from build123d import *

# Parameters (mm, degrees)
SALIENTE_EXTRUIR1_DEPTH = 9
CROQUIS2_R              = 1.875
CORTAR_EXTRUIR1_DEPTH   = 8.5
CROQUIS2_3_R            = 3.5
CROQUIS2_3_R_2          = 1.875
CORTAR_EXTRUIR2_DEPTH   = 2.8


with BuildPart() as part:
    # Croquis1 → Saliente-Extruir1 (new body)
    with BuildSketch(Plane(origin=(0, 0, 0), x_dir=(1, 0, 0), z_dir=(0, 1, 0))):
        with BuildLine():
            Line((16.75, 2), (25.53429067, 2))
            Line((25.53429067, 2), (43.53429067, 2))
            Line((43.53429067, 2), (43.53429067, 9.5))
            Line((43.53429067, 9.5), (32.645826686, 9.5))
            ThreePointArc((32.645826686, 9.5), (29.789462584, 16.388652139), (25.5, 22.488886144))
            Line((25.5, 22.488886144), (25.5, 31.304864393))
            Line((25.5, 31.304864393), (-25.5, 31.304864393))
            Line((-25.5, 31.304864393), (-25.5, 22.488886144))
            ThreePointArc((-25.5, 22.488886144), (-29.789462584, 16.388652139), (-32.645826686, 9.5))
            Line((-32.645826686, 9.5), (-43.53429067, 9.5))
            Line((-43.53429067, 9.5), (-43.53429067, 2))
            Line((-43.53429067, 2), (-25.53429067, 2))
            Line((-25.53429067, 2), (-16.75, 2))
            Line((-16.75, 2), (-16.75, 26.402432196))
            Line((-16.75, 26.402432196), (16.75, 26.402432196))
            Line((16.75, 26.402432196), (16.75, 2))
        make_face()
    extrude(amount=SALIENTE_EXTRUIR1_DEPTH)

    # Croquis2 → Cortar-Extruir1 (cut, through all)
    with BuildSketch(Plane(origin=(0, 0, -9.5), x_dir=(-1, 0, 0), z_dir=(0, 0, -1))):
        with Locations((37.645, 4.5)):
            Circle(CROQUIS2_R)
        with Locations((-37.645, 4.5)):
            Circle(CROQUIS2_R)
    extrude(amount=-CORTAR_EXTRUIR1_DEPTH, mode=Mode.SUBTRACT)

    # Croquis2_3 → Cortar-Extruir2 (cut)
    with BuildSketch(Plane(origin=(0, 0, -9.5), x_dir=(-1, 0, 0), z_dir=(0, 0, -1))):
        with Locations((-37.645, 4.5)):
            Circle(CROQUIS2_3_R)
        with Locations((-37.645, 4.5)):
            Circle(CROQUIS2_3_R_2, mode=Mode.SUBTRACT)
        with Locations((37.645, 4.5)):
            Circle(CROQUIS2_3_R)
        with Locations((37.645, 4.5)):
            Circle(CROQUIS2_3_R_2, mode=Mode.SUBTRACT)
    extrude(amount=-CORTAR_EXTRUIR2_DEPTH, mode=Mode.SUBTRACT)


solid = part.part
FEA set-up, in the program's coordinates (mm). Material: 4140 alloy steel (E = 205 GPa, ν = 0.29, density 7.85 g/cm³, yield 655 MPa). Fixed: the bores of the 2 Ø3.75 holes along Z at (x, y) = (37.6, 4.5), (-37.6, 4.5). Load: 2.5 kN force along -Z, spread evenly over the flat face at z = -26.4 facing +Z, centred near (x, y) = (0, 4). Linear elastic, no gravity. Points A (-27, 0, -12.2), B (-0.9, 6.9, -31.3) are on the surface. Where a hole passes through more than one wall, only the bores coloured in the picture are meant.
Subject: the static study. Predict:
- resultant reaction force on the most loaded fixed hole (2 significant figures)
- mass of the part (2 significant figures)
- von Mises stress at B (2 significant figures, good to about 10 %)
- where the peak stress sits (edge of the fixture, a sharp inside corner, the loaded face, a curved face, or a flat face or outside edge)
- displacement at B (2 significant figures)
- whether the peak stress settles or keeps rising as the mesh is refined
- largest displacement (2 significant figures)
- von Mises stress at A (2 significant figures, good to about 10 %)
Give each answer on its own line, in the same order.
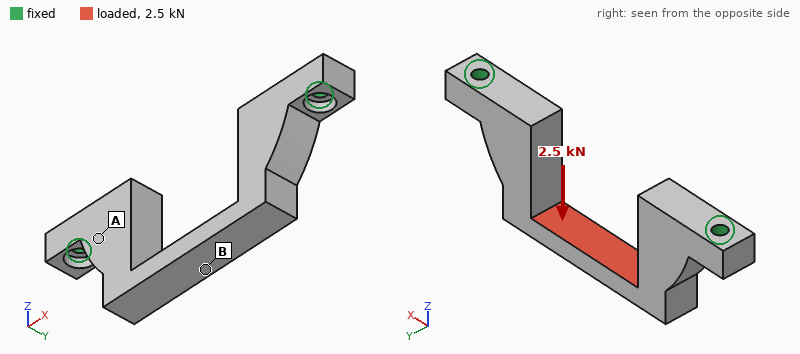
1.7 kN
72 g
160 MPa
edge of the fixture
35 µm
keeps rising
36 µm
23 MPa
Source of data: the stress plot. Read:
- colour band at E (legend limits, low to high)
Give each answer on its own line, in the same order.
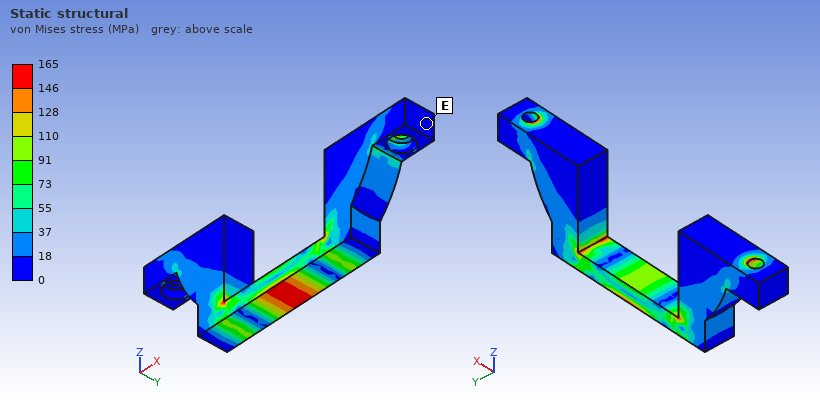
0 to 18 MPa
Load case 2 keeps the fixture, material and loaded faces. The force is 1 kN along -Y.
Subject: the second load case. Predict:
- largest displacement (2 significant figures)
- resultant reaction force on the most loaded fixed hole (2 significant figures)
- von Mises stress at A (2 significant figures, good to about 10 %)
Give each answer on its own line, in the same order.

0.10 mm
500 N
52 MPa
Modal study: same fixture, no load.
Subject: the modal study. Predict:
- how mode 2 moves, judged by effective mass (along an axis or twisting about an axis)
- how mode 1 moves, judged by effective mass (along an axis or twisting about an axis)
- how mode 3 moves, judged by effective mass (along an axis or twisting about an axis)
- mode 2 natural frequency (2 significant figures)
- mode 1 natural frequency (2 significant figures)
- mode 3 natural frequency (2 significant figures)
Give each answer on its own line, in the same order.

along X
along Y
twisting about Z
5100 Hz
3300 Hz
6800 Hz
